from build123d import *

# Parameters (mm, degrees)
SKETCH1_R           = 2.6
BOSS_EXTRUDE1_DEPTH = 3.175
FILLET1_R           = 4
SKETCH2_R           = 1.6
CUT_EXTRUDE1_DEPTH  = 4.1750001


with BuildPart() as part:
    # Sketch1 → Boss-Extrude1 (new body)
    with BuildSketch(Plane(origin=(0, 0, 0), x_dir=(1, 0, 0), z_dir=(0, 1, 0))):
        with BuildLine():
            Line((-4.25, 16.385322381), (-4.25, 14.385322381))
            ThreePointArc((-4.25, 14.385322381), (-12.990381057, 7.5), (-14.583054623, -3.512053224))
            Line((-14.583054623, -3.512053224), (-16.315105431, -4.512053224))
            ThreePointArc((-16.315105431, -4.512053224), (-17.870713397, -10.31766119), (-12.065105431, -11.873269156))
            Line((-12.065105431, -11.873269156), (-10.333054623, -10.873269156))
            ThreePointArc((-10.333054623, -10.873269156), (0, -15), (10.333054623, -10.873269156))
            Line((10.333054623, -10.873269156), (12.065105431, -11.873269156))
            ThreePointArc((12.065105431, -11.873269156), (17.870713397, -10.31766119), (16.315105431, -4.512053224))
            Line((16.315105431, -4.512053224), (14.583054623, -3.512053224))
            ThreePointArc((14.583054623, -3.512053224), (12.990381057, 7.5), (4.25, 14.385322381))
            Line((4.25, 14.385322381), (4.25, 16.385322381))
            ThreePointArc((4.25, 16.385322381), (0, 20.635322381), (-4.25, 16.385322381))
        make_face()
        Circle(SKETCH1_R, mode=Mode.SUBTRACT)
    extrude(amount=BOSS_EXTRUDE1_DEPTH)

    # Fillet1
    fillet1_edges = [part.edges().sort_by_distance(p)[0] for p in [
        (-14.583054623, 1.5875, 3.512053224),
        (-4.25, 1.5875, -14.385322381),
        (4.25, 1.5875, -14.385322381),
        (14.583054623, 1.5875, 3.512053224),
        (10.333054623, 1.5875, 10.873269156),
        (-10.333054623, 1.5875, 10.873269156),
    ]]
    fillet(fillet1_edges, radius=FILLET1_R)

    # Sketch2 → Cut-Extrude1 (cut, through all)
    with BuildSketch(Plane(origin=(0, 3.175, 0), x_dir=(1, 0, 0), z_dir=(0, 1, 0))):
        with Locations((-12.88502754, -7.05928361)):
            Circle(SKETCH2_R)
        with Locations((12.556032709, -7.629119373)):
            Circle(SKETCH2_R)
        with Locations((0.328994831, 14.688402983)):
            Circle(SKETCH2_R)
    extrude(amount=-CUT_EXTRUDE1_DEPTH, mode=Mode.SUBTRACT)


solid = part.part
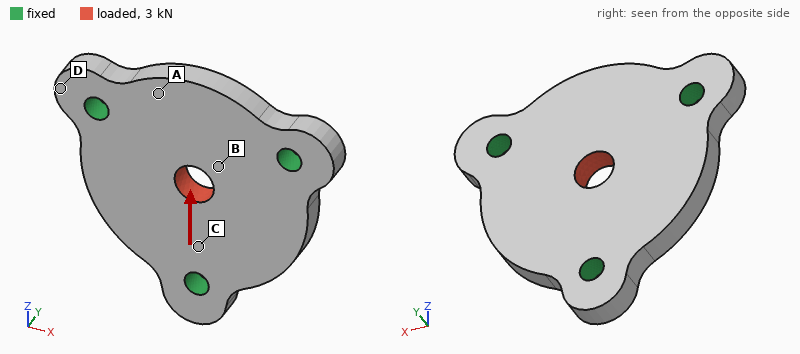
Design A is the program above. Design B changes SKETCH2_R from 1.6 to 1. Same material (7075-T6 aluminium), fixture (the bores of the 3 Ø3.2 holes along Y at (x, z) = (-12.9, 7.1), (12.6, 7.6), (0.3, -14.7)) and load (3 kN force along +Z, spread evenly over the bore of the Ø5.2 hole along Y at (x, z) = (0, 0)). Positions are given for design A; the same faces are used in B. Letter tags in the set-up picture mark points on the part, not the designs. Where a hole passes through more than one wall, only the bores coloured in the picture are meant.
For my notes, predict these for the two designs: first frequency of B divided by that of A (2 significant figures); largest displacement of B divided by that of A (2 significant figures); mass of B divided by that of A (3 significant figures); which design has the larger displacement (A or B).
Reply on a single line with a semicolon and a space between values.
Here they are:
0.87; 1.1; 1.02; B
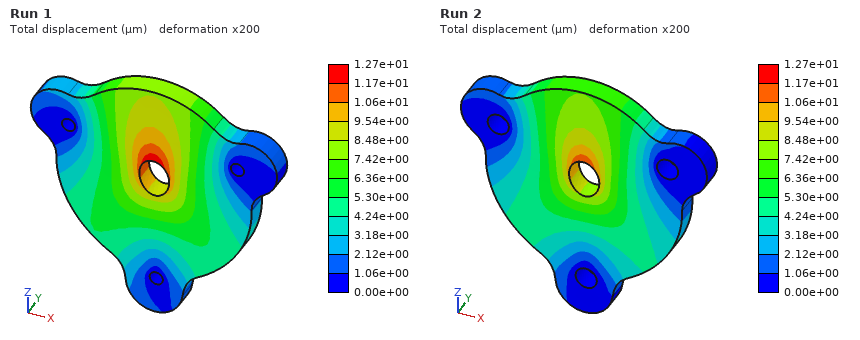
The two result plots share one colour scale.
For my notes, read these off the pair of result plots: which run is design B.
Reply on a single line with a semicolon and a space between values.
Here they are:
Run 1
